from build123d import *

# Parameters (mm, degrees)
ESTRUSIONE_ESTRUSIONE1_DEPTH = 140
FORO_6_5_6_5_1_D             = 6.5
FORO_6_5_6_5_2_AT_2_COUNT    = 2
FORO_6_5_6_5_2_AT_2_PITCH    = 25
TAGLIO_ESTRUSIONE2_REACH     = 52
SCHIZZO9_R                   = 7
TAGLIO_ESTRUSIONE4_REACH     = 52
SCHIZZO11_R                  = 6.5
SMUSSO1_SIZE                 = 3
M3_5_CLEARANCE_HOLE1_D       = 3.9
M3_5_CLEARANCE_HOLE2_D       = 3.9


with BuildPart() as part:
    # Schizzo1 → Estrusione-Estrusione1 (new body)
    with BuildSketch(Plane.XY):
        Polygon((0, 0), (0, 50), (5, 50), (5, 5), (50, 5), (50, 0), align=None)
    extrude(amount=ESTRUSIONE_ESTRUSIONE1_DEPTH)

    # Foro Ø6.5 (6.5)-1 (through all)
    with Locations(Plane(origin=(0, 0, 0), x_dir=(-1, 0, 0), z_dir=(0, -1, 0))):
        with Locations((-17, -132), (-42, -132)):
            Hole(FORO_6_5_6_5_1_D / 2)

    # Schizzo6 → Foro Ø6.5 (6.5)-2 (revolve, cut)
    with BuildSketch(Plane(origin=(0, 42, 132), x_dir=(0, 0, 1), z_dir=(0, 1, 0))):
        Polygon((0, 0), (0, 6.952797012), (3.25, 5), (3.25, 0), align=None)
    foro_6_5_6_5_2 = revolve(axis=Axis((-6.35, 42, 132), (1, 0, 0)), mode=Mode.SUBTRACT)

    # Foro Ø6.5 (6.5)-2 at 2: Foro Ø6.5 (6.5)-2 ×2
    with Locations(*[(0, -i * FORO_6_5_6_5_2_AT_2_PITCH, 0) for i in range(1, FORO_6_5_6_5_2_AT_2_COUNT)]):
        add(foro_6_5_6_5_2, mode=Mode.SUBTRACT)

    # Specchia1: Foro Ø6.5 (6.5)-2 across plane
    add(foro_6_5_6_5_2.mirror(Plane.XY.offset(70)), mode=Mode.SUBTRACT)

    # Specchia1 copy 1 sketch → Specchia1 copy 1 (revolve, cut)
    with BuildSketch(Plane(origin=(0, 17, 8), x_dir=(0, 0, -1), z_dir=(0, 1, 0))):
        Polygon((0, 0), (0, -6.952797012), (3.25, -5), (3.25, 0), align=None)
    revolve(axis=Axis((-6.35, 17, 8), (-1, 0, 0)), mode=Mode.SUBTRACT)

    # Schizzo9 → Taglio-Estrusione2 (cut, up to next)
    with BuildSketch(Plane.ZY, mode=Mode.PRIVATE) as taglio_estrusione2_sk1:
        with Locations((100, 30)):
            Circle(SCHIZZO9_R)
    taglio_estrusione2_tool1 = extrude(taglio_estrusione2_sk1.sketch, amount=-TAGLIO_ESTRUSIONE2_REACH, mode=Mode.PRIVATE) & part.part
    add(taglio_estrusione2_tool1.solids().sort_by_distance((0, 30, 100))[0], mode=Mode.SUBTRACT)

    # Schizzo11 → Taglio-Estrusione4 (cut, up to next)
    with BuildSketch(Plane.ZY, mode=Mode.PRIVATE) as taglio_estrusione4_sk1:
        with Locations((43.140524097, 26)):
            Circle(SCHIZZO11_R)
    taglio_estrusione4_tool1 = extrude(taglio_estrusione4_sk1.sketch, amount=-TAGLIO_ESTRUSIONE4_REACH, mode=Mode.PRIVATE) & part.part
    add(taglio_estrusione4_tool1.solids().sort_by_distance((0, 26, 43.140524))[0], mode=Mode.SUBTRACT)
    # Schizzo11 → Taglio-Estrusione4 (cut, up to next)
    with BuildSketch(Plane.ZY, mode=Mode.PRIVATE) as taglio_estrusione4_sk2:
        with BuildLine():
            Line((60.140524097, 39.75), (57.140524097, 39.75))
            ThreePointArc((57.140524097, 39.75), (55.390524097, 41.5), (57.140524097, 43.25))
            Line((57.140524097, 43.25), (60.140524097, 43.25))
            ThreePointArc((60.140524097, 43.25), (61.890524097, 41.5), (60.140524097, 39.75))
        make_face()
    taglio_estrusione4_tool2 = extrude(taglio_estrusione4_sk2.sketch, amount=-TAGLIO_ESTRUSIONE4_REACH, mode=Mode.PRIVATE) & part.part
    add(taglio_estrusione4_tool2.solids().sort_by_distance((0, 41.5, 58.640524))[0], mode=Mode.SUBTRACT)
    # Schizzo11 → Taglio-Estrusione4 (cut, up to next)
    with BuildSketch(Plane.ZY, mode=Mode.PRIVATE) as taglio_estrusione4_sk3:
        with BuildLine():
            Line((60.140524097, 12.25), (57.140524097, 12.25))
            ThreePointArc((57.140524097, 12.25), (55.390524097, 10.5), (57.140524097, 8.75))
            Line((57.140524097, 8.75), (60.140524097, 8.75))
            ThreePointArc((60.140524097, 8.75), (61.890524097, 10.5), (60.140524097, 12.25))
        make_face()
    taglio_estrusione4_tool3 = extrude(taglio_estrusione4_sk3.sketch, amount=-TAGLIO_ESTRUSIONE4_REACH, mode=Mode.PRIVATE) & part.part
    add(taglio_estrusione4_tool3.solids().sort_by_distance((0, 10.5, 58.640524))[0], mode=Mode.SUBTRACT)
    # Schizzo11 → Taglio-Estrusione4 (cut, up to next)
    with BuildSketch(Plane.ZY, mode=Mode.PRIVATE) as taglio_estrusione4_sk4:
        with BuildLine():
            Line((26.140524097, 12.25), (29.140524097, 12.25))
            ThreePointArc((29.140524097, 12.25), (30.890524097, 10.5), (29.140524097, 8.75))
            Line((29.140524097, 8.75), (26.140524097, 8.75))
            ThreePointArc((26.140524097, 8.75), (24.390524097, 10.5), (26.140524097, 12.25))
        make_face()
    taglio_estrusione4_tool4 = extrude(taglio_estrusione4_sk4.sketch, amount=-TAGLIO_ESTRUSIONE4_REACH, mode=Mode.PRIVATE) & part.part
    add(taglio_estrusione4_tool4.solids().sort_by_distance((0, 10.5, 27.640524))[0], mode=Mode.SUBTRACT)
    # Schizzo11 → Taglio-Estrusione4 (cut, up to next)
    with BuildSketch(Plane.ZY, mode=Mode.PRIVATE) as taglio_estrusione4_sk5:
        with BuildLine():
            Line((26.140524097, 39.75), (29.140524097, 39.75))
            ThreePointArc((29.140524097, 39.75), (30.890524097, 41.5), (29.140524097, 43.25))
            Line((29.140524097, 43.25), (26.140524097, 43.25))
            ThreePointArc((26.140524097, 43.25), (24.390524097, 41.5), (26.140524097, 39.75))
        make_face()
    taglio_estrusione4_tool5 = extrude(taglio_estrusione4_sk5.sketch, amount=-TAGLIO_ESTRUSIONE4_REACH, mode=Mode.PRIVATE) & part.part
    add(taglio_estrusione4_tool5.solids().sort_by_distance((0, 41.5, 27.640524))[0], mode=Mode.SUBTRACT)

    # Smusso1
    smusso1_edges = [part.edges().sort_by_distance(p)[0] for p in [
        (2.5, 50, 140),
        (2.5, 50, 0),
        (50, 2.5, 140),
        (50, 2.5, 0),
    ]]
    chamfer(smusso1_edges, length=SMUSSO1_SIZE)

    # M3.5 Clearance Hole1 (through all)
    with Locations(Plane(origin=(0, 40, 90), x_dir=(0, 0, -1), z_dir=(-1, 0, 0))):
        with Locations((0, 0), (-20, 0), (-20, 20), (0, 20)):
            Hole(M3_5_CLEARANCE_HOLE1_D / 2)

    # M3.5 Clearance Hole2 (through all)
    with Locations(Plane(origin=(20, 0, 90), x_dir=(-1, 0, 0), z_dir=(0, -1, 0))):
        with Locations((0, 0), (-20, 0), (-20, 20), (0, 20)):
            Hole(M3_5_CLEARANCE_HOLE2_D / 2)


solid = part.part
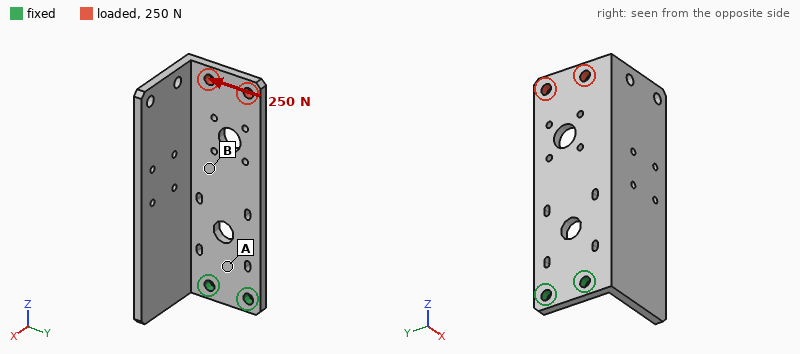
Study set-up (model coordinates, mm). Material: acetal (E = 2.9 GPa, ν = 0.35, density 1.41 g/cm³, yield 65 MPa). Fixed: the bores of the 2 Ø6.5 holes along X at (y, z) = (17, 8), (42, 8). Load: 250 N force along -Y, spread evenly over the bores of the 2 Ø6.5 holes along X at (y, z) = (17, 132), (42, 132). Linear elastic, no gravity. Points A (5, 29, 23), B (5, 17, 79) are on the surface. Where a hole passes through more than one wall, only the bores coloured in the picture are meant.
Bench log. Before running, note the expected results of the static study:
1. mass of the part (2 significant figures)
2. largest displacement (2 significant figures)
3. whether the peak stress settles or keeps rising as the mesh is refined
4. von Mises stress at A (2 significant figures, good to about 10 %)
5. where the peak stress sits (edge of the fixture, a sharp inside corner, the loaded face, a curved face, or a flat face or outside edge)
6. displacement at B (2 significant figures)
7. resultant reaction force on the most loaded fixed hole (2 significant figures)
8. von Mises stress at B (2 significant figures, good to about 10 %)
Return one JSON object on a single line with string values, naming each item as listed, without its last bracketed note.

{"mass of the part": "89 g", "largest displacement": "1.6 mm", "whether the peak stress settles or keeps rising as the mesh is refined": "keeps rising", "von Mises stress at A": "6.1 MPa", "where the peak stress sits": "edge of the fixture", "displacement at B": "0.65 mm", "resultant reaction force on the most loaded fixed hole": "1.1 kN", "von Mises stress at B": "2.4 MPa"}
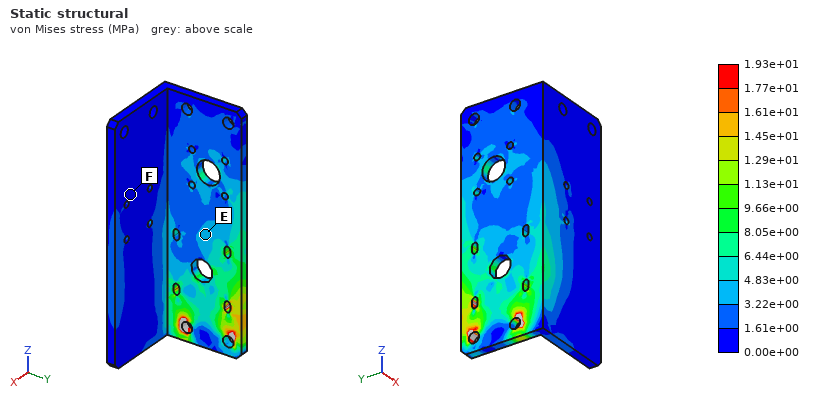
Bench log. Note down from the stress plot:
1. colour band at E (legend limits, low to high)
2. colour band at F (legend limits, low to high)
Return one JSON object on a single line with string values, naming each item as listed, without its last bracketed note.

{"colour band at E": "3.22e+00 to 4.83e+00 MPa", "colour band at F": "0.00e+00 to 1.61e+00 MPa"}
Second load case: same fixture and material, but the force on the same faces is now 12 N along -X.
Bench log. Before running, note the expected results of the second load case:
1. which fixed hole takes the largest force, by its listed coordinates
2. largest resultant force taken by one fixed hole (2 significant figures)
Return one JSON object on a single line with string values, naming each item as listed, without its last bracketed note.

{"which fixed hole takes the largest force, by its listed coordinates": "(17, 8)", "largest resultant force taken by one fixed hole": "12 N"}
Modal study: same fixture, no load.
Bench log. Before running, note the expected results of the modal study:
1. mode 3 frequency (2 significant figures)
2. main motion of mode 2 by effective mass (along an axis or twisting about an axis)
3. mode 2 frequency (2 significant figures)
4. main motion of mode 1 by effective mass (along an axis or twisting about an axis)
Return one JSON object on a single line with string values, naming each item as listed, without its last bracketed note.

{"mode 3 frequency": "420 Hz", "main motion of mode 2 by effective mass": "along Y", "mode 2 frequency": "170 Hz", "main motion of mode 1 by effective mass": "along X"}
